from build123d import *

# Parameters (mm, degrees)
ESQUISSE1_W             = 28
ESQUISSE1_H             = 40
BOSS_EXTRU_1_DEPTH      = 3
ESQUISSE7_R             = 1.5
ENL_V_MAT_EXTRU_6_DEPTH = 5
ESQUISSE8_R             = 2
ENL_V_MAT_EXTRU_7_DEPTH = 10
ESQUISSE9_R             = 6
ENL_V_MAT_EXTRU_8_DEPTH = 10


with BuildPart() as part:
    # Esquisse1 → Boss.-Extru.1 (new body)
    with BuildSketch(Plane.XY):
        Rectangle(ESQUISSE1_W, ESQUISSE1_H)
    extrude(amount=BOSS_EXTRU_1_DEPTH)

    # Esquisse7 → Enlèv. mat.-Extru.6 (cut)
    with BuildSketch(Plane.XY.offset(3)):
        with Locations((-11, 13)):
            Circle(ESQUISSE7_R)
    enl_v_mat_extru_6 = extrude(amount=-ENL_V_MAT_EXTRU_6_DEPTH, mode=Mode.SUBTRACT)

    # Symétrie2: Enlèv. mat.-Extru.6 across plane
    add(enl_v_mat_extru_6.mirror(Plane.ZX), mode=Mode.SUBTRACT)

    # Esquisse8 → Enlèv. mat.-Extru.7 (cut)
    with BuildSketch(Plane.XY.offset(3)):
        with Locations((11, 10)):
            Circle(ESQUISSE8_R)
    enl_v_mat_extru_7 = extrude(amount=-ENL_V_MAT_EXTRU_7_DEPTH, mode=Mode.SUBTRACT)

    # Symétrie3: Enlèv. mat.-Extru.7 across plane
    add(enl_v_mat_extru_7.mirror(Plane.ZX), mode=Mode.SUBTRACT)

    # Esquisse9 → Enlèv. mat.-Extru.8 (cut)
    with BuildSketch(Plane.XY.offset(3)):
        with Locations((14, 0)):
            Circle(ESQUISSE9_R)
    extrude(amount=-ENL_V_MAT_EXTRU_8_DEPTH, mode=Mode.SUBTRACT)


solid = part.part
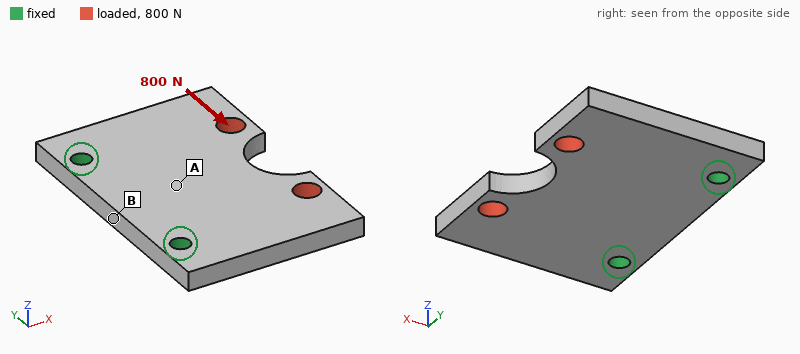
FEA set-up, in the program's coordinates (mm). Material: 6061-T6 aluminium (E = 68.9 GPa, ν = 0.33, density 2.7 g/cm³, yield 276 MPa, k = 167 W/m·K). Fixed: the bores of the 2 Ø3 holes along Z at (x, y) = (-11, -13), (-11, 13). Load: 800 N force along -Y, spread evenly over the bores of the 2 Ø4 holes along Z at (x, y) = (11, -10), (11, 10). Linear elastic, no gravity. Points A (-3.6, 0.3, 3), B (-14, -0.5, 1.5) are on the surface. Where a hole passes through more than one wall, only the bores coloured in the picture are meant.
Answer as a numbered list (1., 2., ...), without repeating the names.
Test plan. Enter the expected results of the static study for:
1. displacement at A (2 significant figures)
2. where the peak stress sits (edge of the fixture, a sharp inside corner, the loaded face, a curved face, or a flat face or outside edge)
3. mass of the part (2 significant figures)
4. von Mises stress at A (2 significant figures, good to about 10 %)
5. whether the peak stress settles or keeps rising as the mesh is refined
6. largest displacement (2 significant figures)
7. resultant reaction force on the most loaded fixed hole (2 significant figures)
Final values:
1. 4.1 µm
2. edge of the fixture
3. 8.3 g
4. 20 MPa
5. keeps rising
6. 18 µm
7. 740 N
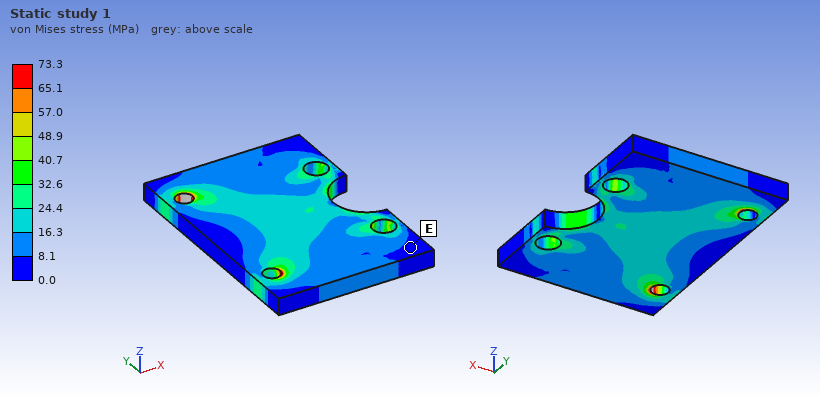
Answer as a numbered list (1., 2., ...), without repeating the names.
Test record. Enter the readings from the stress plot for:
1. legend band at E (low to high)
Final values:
1. 0.0 to 8.1 MPa
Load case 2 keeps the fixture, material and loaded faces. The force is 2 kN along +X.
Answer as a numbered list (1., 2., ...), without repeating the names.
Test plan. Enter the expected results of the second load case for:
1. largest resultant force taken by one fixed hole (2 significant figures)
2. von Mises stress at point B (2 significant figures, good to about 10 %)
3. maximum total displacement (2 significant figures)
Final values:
1. 1.0 kN
2. 13 MPa
3. 15 µm
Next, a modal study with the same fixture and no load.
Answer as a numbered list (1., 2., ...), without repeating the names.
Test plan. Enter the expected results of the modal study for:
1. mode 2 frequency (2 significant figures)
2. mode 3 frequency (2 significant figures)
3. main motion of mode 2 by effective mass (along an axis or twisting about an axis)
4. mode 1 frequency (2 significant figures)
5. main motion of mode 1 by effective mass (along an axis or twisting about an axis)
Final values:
1. 6300 Hz
2. 13 kHz
3. twisting about X
4. 4000 Hz
5. along Z
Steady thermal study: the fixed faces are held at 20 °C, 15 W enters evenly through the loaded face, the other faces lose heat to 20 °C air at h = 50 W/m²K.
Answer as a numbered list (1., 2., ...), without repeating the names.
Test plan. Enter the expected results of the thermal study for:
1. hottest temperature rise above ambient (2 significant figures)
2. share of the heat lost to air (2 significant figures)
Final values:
1. 24 K
2. 8.1 %
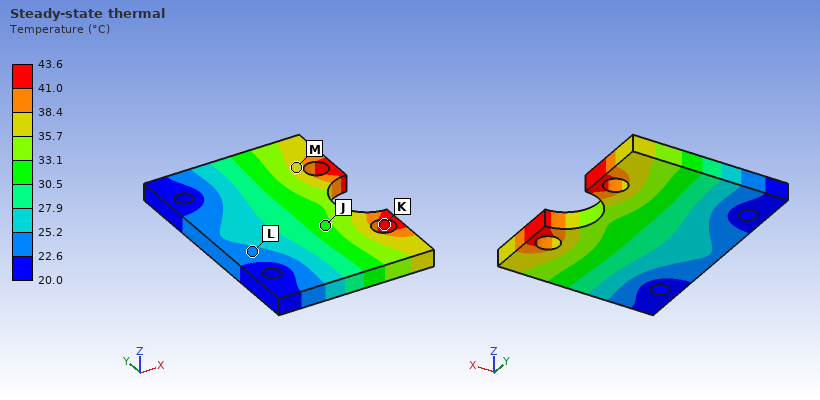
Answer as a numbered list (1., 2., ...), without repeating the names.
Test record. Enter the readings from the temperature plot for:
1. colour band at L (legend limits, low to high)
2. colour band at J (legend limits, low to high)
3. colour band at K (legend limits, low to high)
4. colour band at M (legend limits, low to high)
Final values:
1. 22.6 to 25.2 °C
2. 30.5 to 33.1 °C
3. 41.0 to 43.6 °C
4. 35.7 to 38.4 °C
